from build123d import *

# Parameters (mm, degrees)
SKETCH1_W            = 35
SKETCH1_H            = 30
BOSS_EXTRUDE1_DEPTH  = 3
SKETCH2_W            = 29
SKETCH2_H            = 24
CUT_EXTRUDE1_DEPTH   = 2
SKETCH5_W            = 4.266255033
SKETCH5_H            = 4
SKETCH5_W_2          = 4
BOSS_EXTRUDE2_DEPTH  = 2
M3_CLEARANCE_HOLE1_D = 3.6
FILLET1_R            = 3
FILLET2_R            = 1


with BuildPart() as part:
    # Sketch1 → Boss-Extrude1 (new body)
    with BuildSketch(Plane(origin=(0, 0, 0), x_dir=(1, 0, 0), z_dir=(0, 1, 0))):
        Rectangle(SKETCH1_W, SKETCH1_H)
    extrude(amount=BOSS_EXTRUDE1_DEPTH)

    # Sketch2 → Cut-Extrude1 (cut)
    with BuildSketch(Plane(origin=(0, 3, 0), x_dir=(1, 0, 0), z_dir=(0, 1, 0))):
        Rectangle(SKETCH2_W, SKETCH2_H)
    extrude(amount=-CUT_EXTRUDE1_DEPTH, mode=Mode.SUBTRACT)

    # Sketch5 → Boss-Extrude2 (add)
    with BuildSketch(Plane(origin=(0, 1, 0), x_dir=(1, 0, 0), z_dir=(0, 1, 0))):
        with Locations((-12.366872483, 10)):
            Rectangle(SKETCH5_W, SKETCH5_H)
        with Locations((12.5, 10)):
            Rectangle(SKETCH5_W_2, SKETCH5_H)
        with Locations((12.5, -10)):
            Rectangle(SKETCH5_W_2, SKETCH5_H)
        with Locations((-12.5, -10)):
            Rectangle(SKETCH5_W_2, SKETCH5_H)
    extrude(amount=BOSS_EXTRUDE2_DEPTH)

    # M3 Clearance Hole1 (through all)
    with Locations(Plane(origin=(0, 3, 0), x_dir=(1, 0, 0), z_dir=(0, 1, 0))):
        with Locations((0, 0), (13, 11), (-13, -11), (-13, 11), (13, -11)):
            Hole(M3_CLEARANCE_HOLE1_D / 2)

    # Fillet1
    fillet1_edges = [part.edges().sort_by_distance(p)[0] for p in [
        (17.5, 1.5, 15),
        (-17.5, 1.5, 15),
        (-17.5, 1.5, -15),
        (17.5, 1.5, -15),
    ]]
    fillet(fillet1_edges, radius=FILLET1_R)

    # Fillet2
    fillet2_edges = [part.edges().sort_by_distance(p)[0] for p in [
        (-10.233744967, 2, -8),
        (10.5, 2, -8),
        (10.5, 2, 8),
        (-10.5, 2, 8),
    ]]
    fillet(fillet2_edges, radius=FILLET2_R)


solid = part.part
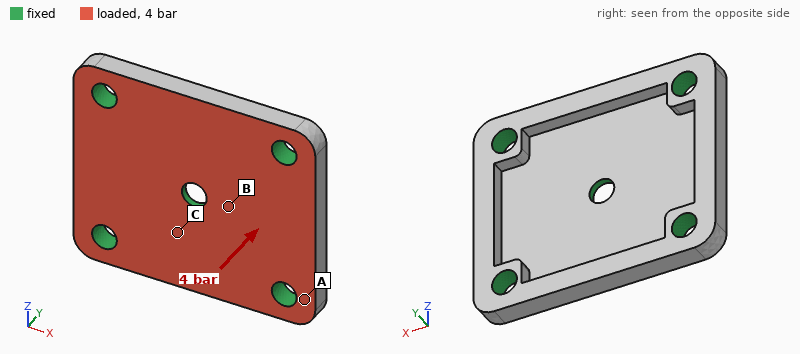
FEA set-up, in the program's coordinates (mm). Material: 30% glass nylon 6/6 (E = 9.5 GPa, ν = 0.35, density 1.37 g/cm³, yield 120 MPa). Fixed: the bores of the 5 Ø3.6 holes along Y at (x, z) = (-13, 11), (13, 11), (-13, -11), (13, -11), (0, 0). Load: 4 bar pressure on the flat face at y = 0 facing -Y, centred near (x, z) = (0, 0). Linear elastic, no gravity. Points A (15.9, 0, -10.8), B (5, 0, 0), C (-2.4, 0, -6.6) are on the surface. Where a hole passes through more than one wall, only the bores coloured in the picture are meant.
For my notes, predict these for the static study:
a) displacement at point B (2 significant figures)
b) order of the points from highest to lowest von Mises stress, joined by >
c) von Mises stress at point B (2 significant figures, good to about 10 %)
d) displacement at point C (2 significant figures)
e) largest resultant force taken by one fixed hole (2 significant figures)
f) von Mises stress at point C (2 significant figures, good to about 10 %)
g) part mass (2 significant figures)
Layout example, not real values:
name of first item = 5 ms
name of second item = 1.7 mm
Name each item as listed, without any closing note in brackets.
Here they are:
displacement at point B = 31 µm
order of the points from highest to lowest von Mises stress, joined by > = C > B > A
von Mises stress at point B = 10 MPa
displacement at point C = 43 µm
largest resultant force taken by one fixed hole = 85 N
von Mises stress at point C = 14 MPa
part mass = 2.4 g
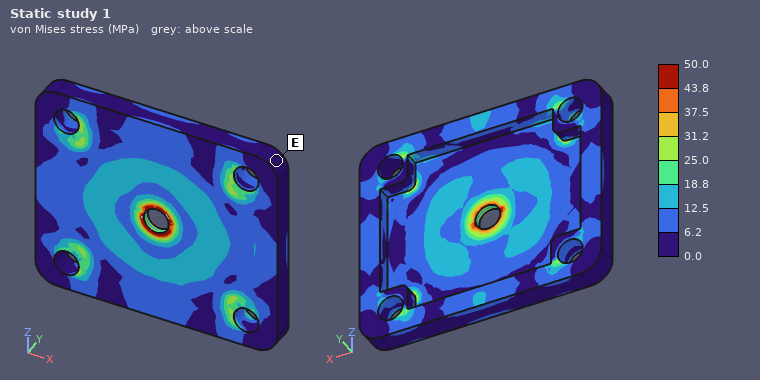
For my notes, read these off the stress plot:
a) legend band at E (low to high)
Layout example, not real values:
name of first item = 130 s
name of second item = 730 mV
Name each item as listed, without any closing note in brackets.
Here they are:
legend band at E = 0.0 to 6.2 MPa
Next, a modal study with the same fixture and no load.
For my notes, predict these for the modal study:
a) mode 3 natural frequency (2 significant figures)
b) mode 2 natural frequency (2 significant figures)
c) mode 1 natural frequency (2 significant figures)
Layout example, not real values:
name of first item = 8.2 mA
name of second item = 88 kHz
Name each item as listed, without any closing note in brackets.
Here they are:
mode 3 natural frequency = 14 kHz
mode 2 natural frequency = 12 kHz
mode 1 natural frequency = 12 kHz
